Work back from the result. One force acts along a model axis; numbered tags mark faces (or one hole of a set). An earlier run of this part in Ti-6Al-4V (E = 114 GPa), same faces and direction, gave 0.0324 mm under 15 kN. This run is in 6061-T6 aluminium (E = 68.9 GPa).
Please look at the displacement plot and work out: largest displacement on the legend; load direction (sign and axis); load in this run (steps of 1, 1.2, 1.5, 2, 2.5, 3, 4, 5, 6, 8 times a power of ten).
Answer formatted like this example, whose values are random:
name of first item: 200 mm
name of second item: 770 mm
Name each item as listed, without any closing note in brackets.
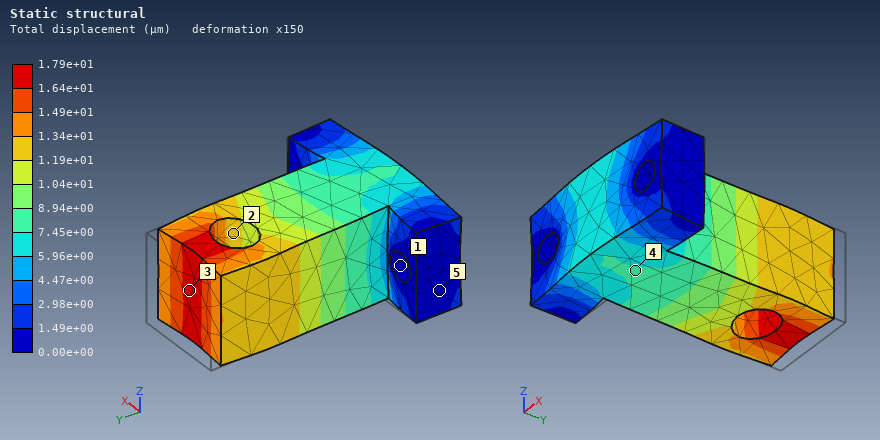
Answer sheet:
largest displacement on the legend: 1.79e+01 µm
load direction: -Y
load in this run: 5 kN
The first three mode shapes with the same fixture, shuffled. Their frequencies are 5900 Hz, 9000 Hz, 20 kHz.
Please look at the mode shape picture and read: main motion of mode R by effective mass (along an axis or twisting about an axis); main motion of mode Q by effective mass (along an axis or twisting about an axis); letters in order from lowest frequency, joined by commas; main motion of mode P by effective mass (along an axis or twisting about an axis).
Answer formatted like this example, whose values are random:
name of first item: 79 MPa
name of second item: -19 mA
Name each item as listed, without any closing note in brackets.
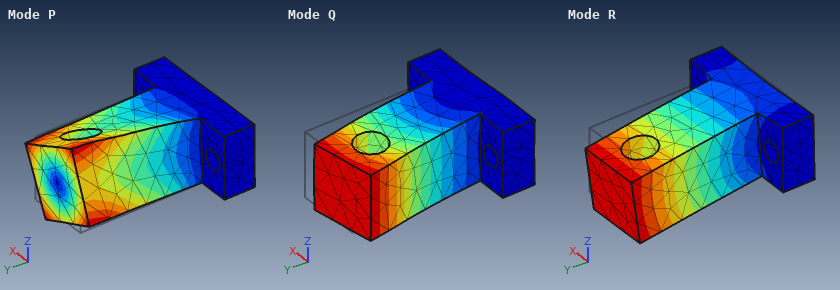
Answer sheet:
main motion of mode R by effective mass: along Z
main motion of mode Q by effective mass: along X
letters in order from lowest frequency, joined by commas: R, Q, P
main motion of mode P by effective mass: twisting about Y
